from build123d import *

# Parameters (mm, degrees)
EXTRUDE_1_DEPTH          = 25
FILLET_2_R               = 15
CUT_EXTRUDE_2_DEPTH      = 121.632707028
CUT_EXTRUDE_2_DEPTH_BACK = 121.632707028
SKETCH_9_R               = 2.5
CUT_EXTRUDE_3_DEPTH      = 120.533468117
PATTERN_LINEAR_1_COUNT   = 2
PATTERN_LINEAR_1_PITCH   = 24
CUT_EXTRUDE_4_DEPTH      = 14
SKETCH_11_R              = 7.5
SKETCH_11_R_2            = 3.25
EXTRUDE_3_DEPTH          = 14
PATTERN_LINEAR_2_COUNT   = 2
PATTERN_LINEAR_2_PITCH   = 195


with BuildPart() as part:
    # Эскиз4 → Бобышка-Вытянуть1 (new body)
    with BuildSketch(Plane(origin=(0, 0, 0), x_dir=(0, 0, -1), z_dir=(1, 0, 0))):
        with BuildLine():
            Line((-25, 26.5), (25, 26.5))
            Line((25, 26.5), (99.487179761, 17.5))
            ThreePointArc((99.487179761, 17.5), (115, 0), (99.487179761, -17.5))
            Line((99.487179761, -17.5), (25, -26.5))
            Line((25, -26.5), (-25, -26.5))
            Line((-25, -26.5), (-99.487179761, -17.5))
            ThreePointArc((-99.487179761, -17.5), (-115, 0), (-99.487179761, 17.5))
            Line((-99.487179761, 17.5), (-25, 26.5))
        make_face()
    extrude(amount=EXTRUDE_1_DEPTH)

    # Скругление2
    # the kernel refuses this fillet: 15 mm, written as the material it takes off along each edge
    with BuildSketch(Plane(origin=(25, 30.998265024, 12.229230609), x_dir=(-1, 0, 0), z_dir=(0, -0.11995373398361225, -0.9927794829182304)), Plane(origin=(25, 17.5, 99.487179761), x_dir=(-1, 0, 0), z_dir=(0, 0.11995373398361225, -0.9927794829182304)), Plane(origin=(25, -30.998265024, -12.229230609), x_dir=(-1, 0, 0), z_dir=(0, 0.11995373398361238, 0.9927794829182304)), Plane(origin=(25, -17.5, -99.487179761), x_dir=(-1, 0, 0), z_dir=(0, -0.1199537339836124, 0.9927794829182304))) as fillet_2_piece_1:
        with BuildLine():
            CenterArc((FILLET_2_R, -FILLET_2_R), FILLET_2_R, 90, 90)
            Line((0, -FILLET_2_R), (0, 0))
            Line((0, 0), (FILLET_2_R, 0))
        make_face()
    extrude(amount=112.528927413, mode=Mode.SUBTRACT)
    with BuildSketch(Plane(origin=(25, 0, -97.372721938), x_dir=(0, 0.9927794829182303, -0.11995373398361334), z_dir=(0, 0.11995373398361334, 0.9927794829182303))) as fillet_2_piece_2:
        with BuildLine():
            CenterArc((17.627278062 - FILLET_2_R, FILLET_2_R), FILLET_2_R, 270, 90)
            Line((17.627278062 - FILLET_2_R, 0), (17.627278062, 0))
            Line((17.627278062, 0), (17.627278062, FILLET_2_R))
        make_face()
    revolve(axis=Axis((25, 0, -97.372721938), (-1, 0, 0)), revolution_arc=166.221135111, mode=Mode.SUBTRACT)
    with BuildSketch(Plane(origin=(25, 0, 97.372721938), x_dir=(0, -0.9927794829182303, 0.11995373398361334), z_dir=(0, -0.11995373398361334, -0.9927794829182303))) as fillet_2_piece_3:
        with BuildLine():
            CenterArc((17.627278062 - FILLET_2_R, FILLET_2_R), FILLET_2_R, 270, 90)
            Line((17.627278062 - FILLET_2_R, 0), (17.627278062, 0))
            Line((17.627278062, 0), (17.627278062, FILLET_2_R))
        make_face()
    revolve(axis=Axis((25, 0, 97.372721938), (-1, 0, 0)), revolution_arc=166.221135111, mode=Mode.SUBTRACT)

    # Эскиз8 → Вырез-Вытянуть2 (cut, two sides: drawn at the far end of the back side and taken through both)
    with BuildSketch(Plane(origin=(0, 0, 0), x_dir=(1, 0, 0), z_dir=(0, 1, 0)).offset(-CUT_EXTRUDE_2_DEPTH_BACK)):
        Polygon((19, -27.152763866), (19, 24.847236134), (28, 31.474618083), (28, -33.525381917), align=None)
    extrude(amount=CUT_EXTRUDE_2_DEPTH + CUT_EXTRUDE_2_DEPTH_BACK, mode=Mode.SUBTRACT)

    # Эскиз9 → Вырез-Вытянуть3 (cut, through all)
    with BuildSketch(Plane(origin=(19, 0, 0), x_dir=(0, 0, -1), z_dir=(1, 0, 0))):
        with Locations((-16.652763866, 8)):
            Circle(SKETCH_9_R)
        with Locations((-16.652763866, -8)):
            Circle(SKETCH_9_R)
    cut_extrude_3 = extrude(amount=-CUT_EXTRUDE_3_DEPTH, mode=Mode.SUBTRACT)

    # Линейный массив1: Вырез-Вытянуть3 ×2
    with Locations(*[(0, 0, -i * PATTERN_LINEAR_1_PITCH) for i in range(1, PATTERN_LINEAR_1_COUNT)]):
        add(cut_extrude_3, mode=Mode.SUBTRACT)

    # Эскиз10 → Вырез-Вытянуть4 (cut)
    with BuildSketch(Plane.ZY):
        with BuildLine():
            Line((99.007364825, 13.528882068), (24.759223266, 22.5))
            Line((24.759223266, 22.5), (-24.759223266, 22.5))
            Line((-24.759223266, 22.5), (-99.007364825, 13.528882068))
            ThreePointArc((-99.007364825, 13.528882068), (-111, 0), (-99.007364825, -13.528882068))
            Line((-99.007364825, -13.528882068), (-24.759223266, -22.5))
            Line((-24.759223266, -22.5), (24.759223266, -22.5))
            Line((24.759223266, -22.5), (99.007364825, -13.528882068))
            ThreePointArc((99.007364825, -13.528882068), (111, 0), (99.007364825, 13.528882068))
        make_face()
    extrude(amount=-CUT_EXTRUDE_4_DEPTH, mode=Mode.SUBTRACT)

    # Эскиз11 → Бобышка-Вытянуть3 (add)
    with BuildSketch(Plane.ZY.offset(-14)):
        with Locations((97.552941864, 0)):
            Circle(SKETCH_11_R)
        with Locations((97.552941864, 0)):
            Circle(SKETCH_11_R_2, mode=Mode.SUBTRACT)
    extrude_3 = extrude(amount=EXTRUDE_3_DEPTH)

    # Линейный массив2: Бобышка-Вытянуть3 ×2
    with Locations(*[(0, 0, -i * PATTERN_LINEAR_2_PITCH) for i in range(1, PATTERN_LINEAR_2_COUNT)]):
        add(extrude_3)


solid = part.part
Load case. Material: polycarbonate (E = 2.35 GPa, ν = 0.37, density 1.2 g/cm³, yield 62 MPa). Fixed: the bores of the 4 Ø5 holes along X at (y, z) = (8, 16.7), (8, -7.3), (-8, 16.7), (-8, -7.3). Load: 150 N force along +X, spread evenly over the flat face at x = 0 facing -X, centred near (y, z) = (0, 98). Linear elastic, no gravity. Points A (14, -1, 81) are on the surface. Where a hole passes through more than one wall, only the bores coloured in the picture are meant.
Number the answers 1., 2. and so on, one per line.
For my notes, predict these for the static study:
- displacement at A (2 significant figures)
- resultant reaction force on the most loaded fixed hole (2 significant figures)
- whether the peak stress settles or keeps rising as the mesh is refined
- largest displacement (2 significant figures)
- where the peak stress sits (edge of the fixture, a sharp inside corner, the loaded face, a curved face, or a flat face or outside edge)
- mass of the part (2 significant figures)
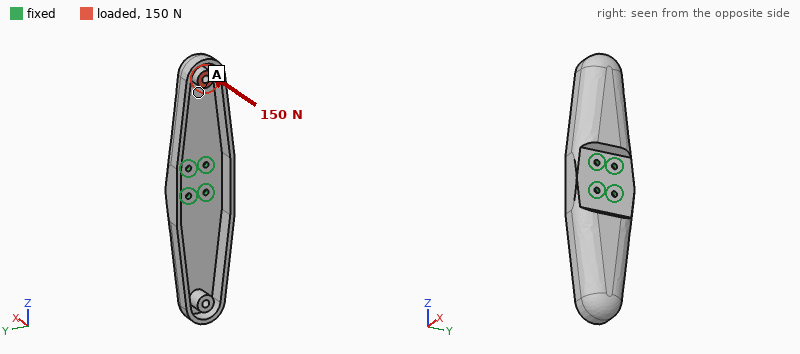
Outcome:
1. 1.7 mm
2. 250 N
3. keeps rising
4. 2.8 mm
5. edge of the fixture
6. 130 g
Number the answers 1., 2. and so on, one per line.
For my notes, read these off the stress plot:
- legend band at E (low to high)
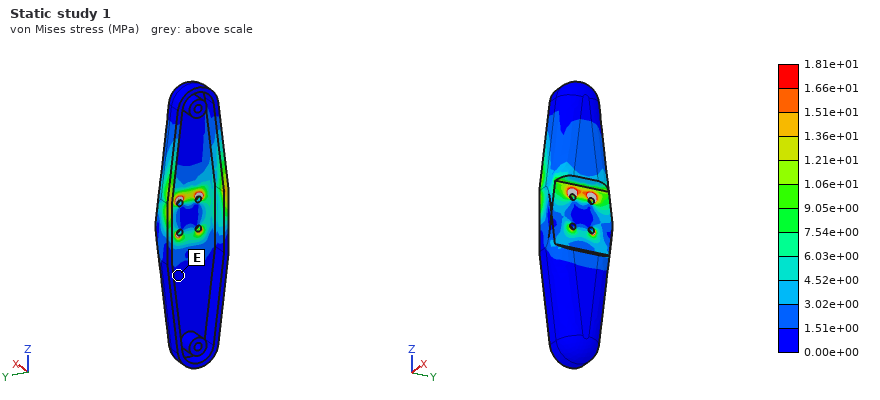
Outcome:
1. 0.00e+00 to 1.51e+00 MPa
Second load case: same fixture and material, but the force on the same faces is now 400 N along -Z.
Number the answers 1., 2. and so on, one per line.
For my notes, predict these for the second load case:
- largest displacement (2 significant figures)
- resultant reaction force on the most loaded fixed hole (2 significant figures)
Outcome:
1. 1.8 mm
2. 150 N
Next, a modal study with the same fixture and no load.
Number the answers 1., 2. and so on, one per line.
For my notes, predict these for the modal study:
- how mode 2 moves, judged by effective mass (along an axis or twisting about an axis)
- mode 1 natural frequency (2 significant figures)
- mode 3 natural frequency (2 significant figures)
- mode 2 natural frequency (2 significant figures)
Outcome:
1. along X
2. 200 Hz
3. 570 Hz
4. 300 Hz
